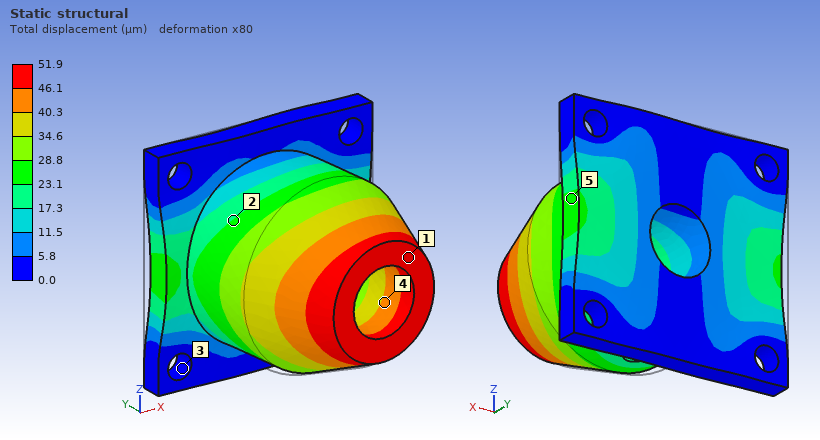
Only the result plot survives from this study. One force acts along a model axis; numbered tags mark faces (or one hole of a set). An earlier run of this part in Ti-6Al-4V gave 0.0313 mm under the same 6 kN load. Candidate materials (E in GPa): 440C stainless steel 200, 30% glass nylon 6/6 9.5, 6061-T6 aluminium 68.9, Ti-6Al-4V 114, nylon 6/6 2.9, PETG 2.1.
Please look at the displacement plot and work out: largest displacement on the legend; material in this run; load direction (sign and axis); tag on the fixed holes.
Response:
51.9 µm
6061-T6 aluminium
+X
3
